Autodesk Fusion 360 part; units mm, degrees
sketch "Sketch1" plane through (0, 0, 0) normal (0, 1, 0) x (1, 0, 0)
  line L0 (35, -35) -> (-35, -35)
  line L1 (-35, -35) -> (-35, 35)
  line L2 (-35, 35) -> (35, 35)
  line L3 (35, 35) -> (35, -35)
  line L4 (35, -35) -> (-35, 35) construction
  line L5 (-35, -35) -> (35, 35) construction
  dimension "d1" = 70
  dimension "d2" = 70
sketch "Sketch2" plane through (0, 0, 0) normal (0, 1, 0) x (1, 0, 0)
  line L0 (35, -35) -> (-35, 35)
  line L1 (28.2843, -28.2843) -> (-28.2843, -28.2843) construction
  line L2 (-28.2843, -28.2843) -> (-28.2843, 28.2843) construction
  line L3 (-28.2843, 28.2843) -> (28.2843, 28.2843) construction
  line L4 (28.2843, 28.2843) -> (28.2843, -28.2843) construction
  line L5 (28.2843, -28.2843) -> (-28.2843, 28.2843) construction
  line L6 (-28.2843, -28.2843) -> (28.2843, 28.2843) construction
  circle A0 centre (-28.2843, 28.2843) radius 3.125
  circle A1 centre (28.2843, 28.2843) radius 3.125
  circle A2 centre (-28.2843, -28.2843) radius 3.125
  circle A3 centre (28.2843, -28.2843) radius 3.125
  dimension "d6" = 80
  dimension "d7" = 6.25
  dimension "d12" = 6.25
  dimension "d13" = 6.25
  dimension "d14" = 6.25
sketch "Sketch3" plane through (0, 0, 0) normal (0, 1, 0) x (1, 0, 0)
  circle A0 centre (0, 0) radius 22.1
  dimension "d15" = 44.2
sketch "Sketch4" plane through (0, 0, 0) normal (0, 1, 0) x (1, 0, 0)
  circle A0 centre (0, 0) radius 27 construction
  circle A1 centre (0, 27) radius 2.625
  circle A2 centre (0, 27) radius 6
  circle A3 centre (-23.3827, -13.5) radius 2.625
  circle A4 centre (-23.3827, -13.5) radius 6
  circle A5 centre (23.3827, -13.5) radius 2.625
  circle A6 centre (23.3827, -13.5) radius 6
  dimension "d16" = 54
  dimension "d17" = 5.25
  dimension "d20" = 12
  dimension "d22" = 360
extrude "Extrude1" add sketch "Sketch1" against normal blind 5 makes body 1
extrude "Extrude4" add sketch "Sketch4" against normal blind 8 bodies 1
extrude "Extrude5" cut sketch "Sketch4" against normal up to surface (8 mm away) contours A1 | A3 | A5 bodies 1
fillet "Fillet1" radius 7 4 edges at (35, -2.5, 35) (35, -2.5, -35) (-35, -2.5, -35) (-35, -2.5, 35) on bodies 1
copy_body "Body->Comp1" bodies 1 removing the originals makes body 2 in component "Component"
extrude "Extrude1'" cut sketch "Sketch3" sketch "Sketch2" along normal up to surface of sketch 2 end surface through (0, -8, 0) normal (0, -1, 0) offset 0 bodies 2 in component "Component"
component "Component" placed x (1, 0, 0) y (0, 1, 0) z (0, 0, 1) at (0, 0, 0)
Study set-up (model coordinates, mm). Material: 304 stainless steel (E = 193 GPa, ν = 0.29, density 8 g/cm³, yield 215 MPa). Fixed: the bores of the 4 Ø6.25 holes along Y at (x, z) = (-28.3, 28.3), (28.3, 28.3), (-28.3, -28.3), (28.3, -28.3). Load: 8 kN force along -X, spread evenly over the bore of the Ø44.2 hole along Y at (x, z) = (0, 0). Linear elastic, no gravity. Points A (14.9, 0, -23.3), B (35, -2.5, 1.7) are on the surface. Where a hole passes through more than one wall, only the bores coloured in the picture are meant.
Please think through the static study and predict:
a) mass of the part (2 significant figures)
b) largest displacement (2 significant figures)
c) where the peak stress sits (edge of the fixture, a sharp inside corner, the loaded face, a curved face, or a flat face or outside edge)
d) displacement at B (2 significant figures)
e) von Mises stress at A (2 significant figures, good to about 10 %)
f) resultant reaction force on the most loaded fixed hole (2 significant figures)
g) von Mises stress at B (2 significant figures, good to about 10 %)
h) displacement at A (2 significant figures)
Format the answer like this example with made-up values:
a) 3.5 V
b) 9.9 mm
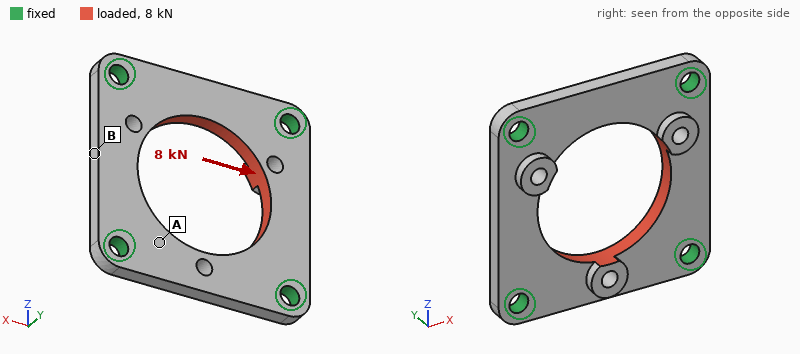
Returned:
a) 130 g
b) 7.7 µm
c) edge of the fixture
d) 7.1 µm
e) 19 MPa
f) 2.1 kN
g) 36 MPa
h) 2.5 µm
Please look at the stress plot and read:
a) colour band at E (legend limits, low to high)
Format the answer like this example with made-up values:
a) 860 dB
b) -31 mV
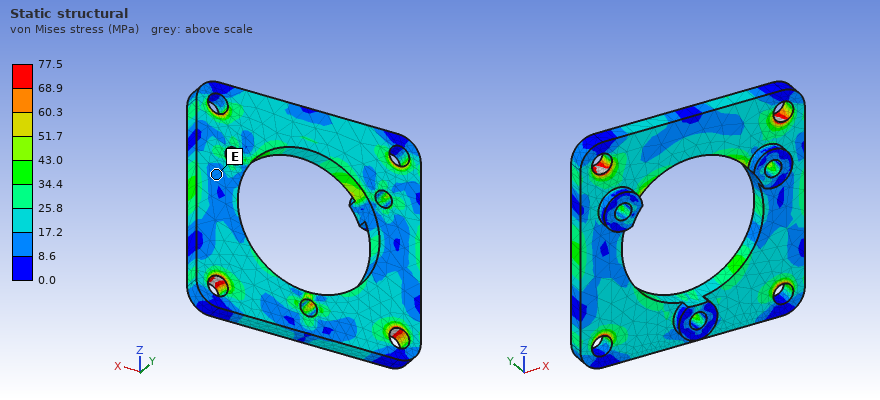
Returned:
a) 8.6 to 17.2 MPa
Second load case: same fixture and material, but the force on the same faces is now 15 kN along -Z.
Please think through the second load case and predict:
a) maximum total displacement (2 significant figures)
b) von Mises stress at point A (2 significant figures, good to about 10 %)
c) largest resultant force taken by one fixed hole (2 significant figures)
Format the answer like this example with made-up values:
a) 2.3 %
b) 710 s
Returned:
a) 17 µm
b) 29 MPa
c) 3.8 kN
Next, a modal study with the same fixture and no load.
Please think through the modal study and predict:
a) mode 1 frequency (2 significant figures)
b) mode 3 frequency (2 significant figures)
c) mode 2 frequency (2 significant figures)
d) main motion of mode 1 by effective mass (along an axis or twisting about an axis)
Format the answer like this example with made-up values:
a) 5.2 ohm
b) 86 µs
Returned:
a) 8500 Hz
b) 9000 Hz
c) 8900 Hz
d) along Y
